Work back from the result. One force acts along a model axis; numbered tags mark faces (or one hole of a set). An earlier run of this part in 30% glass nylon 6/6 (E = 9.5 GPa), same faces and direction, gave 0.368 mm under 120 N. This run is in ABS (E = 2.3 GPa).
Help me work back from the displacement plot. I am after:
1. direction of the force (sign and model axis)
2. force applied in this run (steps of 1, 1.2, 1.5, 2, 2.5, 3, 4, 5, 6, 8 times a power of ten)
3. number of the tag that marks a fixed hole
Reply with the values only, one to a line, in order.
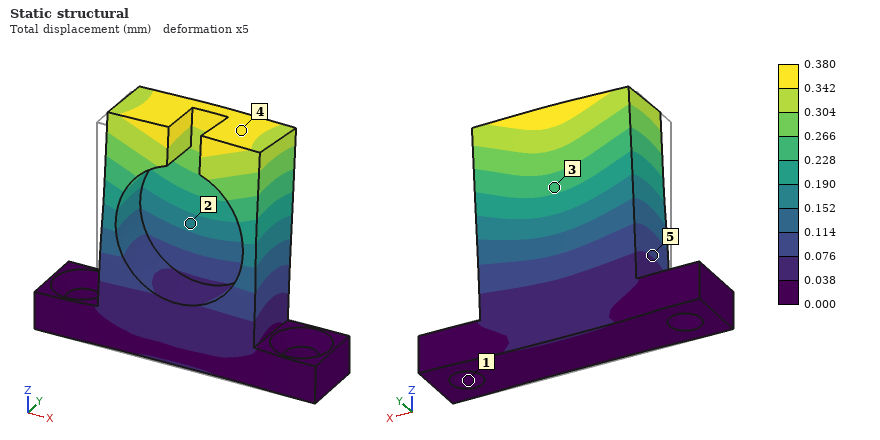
+Y
30 N
1
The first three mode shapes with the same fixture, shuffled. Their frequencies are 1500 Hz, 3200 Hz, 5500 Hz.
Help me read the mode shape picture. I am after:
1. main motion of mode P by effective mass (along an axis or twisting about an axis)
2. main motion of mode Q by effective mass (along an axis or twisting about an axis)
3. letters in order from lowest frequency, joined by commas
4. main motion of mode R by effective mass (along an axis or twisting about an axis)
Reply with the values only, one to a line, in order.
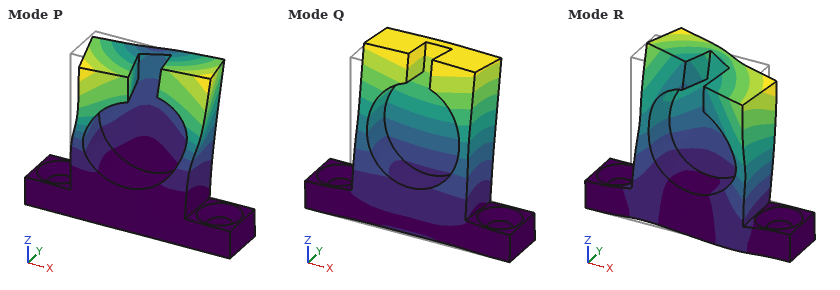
along X
along Y
Q, P, R
along X
